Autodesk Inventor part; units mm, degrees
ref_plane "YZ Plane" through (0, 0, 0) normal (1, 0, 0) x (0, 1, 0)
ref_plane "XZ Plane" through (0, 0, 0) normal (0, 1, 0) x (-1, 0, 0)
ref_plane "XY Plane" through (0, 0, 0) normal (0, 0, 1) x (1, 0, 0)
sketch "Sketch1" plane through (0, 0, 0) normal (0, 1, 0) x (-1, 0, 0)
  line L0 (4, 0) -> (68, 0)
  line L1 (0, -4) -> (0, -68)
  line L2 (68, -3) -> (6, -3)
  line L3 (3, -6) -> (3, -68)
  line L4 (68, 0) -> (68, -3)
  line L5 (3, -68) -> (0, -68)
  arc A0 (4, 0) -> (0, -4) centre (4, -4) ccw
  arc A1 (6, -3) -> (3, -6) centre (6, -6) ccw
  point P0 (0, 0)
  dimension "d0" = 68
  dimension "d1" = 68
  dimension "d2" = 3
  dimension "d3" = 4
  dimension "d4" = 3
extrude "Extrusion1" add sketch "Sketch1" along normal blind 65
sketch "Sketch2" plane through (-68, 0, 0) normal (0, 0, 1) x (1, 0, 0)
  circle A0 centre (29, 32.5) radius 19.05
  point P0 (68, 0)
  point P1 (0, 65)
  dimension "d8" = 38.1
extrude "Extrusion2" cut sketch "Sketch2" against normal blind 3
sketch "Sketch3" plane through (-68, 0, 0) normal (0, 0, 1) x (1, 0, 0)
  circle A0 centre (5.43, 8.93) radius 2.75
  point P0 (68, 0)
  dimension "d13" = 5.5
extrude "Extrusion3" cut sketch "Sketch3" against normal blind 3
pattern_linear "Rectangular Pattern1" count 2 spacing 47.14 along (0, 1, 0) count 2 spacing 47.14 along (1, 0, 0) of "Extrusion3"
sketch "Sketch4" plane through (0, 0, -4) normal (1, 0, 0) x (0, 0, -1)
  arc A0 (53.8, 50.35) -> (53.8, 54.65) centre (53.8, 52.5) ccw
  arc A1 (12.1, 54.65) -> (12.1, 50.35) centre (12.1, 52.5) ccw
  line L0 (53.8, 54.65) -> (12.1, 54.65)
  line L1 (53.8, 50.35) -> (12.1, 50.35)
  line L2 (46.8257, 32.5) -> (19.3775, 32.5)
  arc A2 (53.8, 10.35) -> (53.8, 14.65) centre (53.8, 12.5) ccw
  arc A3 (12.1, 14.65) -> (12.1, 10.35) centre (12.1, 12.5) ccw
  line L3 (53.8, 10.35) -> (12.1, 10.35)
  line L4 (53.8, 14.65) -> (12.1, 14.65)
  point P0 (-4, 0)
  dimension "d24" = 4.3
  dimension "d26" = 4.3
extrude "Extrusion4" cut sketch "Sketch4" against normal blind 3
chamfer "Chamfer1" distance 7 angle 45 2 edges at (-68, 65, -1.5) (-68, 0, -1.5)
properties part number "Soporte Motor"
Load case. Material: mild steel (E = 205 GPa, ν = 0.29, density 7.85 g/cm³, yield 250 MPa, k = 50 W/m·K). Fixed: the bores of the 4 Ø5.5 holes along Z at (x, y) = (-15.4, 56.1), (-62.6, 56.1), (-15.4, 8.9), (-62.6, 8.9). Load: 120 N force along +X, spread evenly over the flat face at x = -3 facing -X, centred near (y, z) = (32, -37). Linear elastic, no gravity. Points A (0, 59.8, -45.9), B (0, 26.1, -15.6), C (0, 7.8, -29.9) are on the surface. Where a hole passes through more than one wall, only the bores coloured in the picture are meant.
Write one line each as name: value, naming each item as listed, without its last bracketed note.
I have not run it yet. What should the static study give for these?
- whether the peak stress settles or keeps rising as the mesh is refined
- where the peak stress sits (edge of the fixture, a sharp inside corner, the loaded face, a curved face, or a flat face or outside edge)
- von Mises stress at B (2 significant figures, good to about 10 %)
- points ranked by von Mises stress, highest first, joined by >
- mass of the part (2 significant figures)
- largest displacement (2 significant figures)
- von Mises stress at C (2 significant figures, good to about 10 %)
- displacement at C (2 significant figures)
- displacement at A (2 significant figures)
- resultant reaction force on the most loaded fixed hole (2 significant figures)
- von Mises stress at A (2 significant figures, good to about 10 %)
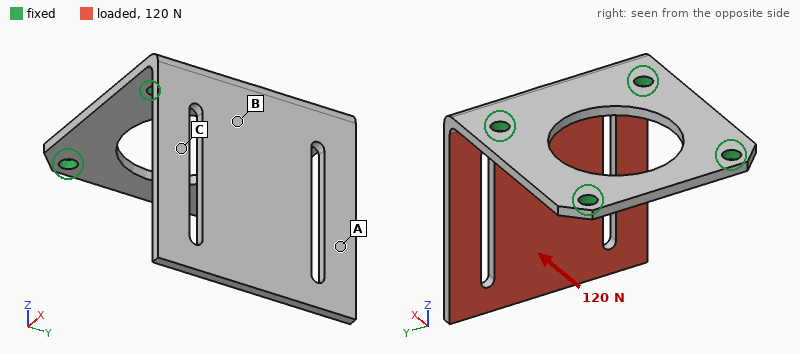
whether the peak stress settles or keeps rising as the mesh is refined: keeps rising
where the peak stress sits: edge of the fixture
von Mises stress at B: 27 MPa
points ranked by von Mises stress, highest first, joined by >: B > C > A
mass of the part: 160 g
largest displacement: 0.27 mm
von Mises stress at C: 17 MPa
displacement at C: 0.088 mm
displacement at A: 0.16 mm
resultant reaction force on the most loaded fixed hole: 63 N
von Mises stress at A: 6.4 MPa
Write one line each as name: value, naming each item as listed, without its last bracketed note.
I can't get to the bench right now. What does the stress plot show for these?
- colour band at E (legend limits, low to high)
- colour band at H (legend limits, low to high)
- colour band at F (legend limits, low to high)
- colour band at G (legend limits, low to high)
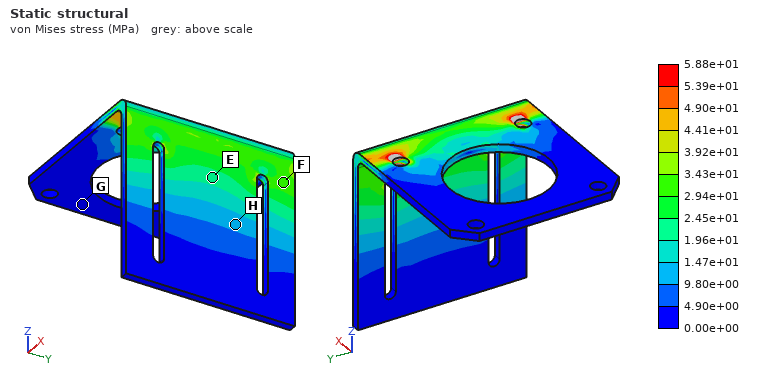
colour band at E: 1.96e+01 to 2.45e+01 MPa
colour band at H: 9.80e+00 to 1.47e+01 MPa
colour band at F: 2.94e+01 to 3.43e+01 MPa
colour band at G: 0.00e+00 to 4.90e+00 MPa
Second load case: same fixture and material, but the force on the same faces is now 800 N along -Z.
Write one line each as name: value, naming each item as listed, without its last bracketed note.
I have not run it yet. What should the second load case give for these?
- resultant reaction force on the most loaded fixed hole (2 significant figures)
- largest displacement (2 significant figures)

resultant reaction force on the most loaded fixed hole: 410 N
largest displacement: 83 µm
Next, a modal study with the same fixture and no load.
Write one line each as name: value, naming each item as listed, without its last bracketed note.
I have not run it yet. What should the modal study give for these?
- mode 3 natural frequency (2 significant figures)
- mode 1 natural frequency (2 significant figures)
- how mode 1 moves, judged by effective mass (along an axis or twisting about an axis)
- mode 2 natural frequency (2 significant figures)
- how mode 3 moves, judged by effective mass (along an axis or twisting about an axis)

mode 3 natural frequency: 2100 Hz
mode 1 natural frequency: 450 Hz
how mode 1 moves, judged by effective mass: along X
mode 2 natural frequency: 1200 Hz
how mode 3 moves, judged by effective mass: along Y
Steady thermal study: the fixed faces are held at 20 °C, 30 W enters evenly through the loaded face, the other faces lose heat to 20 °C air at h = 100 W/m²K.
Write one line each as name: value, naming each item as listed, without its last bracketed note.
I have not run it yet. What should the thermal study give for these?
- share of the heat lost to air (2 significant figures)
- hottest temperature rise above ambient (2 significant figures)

share of the heat lost to air: 74 %
hottest temperature rise above ambient: 49 K
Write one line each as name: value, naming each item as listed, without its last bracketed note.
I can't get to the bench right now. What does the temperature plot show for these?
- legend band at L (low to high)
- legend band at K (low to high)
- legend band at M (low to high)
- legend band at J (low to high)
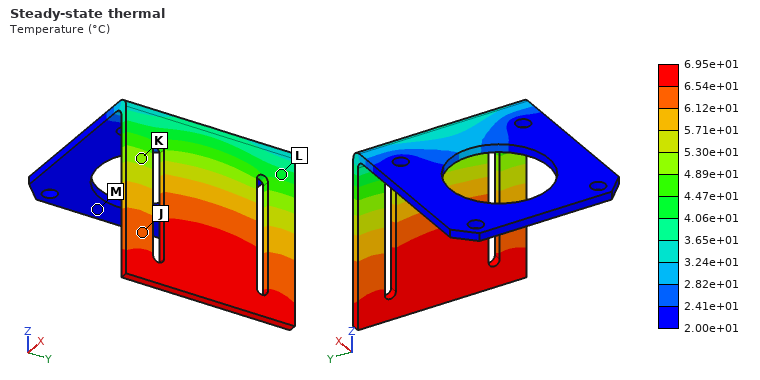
legend band at L: 4.06e+01 to 4.47e+01 °C
legend band at K: 4.89e+01 to 5.30e+01 °C
legend band at M: 2.00e+01 to 2.41e+01 °C
legend band at J: 6.12e+01 to 6.54e+01 °C
